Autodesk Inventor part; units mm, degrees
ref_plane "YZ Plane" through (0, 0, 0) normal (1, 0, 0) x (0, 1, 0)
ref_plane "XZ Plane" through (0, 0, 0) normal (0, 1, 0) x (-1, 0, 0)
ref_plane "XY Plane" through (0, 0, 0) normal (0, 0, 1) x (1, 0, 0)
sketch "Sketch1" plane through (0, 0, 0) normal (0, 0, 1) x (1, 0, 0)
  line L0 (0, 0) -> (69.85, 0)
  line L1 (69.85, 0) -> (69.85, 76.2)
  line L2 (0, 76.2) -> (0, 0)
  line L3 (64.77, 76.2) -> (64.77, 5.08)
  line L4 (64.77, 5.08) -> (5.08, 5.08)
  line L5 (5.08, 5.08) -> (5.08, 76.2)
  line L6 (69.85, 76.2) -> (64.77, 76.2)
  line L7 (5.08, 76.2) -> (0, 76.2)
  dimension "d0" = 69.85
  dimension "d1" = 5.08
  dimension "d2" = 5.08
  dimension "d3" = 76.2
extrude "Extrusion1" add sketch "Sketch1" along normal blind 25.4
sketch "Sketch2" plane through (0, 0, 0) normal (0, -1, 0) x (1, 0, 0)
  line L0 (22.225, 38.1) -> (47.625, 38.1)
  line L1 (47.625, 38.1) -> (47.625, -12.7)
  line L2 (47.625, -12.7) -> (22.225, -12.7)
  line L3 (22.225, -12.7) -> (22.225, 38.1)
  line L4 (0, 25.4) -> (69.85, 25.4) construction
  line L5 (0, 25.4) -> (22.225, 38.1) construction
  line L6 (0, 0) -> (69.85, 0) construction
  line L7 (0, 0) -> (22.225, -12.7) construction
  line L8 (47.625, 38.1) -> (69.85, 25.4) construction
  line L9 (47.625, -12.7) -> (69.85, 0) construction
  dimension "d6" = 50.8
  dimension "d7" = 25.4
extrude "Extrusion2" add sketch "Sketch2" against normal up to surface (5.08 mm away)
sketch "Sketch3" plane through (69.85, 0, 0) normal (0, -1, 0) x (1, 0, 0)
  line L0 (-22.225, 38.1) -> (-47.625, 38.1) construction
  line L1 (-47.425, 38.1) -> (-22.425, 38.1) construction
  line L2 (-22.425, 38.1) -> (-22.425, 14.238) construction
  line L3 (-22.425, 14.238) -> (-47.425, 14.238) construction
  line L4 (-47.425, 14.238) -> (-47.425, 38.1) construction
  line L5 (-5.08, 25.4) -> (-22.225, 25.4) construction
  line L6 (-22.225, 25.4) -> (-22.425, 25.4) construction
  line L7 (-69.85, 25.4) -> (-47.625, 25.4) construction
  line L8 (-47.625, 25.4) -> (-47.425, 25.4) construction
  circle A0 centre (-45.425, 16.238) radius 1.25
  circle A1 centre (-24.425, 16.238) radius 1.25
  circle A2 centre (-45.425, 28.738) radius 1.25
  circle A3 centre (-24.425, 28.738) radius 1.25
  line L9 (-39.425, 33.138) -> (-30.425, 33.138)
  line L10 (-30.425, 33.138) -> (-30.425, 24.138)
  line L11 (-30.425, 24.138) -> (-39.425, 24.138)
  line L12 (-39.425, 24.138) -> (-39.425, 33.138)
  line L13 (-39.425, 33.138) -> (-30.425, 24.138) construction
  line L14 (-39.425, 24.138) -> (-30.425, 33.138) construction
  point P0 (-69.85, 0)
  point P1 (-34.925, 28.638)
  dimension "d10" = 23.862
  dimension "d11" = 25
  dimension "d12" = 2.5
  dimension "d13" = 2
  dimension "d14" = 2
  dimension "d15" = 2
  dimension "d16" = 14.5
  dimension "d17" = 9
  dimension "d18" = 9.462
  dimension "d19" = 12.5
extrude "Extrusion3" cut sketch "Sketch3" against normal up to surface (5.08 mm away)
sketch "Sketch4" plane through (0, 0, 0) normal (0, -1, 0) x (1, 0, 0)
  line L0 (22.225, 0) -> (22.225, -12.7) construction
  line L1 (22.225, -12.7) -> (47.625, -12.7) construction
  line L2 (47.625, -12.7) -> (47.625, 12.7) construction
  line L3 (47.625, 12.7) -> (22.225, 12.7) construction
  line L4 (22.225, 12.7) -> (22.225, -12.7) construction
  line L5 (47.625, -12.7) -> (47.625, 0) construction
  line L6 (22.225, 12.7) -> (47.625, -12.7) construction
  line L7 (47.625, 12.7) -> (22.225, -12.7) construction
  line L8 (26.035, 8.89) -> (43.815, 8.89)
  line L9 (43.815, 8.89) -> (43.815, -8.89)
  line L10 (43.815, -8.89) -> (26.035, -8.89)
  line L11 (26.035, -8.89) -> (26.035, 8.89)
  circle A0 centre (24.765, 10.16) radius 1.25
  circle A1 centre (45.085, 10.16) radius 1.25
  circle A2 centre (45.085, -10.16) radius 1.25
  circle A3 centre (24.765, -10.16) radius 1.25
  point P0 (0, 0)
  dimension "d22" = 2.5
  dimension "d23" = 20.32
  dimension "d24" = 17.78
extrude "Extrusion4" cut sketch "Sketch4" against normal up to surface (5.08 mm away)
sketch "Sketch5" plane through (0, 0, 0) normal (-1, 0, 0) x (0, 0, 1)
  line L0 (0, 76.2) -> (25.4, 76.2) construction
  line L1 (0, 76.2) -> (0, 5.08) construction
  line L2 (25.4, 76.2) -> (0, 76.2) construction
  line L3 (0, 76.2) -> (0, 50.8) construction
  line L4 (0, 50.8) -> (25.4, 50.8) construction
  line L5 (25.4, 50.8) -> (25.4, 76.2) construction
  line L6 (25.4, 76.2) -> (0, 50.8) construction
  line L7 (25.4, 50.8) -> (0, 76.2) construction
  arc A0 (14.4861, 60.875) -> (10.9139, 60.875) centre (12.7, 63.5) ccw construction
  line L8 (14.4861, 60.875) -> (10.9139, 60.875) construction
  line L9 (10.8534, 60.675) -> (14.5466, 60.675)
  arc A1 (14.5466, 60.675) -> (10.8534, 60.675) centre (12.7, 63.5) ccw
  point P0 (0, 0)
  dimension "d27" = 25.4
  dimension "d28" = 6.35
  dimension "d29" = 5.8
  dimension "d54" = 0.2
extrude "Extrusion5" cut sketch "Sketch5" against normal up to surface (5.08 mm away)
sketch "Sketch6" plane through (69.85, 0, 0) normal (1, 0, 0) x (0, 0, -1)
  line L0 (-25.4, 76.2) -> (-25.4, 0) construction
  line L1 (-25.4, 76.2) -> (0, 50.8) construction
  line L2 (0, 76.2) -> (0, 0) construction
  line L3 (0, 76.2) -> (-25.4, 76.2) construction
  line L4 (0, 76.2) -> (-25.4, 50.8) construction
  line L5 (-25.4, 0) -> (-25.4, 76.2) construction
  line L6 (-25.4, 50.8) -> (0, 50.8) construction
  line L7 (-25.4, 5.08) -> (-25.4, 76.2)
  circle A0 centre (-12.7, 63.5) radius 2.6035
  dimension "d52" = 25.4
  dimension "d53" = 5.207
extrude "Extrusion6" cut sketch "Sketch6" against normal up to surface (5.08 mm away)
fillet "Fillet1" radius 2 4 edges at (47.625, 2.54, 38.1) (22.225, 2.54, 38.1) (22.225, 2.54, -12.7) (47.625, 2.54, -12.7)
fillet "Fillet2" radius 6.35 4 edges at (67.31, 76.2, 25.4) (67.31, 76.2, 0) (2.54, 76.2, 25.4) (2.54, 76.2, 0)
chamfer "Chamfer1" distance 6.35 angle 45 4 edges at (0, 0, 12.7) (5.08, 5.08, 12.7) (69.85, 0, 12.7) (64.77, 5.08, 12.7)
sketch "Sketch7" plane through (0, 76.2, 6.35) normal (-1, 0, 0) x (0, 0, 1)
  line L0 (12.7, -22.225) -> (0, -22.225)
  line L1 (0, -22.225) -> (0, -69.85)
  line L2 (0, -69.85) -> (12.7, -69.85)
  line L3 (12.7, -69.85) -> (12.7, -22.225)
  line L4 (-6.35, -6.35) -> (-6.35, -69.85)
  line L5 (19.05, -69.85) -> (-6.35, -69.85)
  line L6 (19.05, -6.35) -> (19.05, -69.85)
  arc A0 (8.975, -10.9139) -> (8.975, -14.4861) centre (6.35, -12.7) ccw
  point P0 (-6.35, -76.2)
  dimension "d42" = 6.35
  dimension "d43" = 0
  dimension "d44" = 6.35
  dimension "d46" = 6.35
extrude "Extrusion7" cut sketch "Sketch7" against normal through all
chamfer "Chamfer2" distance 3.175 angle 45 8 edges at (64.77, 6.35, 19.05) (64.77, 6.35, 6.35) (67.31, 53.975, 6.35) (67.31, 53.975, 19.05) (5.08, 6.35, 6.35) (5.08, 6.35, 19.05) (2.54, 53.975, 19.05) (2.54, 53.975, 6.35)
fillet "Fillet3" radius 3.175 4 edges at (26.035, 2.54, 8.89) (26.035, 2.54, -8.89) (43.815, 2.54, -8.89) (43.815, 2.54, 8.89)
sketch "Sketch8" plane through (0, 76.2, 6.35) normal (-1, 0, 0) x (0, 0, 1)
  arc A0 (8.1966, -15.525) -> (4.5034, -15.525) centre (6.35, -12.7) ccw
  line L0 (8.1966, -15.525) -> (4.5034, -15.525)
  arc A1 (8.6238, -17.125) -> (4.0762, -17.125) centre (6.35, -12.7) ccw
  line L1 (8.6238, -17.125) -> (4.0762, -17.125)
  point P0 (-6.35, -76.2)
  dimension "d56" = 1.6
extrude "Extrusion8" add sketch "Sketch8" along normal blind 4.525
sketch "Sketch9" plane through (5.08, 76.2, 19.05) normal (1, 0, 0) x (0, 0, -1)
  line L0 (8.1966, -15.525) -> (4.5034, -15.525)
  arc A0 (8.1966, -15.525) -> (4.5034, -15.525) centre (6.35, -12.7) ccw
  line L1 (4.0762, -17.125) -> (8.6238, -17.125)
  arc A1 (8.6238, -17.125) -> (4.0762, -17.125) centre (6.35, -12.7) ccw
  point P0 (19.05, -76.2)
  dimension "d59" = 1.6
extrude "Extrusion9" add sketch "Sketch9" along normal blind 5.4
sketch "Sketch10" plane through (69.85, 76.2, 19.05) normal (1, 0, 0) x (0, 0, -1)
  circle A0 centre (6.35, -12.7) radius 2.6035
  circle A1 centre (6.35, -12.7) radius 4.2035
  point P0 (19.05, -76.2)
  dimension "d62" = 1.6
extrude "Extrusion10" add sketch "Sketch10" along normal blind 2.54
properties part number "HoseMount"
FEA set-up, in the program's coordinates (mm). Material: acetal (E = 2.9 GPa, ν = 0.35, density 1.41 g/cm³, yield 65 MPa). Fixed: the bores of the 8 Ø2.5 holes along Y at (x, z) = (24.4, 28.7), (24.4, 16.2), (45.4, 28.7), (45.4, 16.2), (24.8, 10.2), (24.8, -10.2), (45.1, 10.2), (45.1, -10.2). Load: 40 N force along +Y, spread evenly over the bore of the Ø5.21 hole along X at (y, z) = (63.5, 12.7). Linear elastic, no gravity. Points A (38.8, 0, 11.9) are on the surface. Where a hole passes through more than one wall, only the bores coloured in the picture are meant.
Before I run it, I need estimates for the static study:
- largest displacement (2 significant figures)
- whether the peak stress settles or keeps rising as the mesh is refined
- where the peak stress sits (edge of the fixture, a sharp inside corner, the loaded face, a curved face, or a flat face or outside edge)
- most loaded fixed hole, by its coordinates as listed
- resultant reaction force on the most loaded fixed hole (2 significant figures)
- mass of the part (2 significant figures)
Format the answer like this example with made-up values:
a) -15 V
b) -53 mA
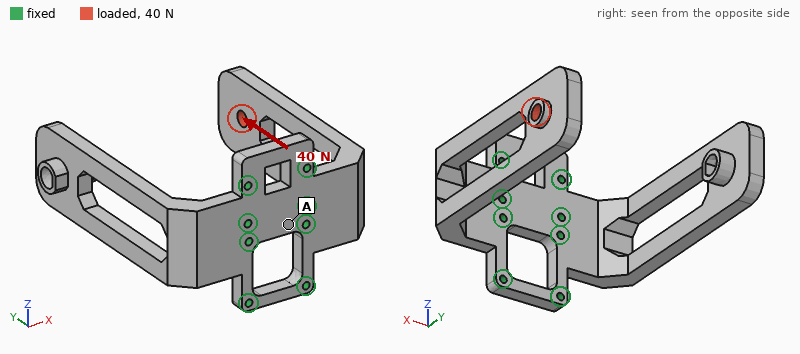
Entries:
a) 1.3 mm
b) keeps rising
c) edge of the fixture
d) (45.4, 16.2)
e) 33 N
f) 31 g
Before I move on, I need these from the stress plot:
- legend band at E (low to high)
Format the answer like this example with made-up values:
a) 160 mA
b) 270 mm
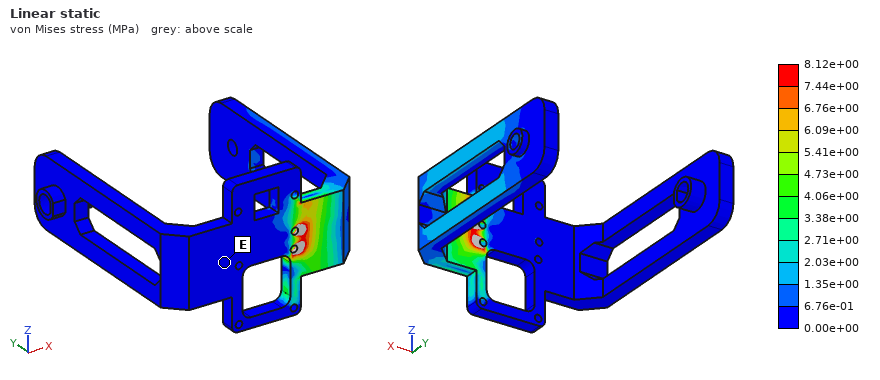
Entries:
a) 0.00e+00 to 6.76e-01 MPa
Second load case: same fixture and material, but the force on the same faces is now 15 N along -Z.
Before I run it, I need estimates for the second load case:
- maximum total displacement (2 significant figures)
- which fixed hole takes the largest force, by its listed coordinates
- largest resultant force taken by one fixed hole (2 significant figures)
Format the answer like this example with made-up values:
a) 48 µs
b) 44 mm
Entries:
a) 1.1 mm
b) (45.1, 10.2)
c) 43 N
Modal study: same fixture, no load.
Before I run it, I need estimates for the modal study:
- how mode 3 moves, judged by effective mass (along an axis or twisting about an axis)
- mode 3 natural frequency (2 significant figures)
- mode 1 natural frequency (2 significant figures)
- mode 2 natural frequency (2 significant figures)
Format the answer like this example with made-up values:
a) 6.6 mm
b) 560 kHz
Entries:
a) along Z
b) 260 Hz
c) 150 Hz
d) 150 Hz
